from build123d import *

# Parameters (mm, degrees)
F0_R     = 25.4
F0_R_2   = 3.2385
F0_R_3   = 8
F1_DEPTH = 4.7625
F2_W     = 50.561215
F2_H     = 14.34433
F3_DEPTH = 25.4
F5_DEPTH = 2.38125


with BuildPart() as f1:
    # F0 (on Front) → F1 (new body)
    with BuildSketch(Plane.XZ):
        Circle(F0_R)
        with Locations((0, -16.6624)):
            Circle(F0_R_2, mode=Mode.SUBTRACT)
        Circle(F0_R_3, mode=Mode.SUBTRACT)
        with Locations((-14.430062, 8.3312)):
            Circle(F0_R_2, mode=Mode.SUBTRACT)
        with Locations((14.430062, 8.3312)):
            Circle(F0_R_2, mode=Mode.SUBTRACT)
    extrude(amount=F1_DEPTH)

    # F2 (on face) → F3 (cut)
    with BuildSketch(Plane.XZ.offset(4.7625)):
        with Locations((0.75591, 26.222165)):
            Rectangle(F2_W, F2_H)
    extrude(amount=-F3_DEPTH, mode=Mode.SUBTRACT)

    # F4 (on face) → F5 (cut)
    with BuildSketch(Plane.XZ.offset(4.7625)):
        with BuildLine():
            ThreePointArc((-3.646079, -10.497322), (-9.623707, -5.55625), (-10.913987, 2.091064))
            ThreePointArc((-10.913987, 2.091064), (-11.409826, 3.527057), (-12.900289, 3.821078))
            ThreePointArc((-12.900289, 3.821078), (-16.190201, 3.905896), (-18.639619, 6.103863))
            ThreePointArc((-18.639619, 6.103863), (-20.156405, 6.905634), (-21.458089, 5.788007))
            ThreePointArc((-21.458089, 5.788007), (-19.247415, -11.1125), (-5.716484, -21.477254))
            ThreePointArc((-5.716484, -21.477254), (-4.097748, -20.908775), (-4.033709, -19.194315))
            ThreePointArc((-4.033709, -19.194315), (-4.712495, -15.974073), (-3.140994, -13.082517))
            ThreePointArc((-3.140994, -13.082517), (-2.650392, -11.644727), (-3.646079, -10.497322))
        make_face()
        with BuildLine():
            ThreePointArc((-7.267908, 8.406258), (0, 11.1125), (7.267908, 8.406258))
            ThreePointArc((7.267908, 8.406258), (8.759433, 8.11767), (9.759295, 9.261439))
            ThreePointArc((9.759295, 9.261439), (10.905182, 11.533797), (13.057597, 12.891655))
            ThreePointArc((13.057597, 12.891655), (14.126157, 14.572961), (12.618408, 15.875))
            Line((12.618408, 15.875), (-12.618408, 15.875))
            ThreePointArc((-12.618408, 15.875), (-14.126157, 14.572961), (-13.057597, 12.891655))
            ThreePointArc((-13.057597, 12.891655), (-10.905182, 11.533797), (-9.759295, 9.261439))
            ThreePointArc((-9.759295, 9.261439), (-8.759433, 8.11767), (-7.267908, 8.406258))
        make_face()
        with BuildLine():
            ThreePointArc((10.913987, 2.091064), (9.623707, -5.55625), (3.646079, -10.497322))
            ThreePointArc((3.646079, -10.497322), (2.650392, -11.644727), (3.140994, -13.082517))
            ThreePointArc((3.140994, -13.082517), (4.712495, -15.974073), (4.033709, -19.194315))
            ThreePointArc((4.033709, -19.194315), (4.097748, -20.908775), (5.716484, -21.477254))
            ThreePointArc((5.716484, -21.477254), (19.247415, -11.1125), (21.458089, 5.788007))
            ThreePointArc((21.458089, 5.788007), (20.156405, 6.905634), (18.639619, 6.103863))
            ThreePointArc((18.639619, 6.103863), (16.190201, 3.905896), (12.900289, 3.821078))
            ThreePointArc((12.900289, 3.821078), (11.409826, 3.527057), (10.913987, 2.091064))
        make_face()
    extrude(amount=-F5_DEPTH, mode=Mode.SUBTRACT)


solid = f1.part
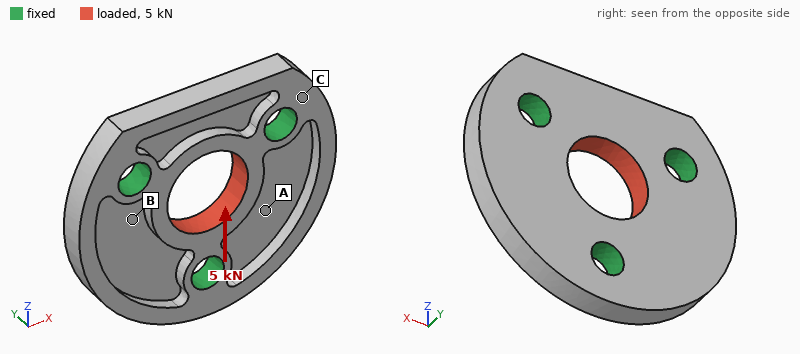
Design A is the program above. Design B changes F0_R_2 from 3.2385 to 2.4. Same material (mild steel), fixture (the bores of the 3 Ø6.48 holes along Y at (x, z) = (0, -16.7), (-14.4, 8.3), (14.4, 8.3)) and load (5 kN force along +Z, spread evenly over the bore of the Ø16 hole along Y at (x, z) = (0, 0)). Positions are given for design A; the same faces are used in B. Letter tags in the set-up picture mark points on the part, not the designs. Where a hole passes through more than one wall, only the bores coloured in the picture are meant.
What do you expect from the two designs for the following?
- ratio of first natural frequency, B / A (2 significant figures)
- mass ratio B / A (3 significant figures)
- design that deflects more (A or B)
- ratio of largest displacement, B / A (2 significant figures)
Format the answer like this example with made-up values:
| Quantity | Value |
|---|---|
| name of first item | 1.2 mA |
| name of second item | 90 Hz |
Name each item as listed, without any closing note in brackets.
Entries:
| Quantity | Value |
|---|---|
| ratio of first natural frequency, B / A | 0.94 |
| mass ratio B / A | 1.04 |
| design that deflects more | B |
| ratio of largest displacement, B / A | 1.1 |
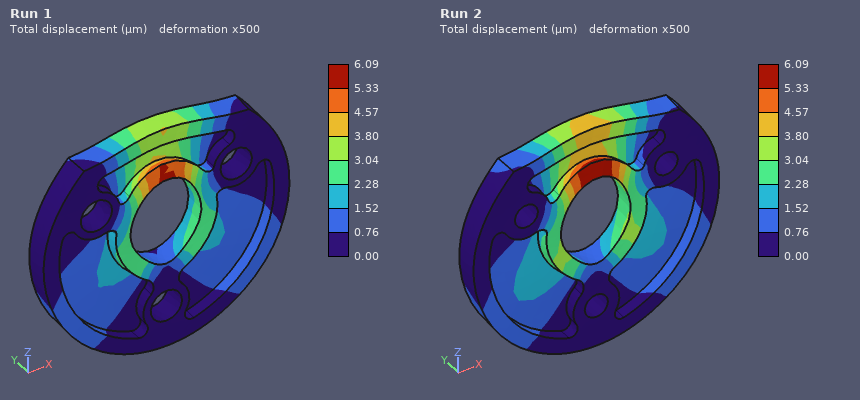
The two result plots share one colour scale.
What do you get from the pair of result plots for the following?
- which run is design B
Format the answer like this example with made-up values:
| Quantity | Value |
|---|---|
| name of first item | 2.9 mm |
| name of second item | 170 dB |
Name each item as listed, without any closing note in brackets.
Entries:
| Quantity | Value |
|---|---|
| which run is design B | Run 2 |
